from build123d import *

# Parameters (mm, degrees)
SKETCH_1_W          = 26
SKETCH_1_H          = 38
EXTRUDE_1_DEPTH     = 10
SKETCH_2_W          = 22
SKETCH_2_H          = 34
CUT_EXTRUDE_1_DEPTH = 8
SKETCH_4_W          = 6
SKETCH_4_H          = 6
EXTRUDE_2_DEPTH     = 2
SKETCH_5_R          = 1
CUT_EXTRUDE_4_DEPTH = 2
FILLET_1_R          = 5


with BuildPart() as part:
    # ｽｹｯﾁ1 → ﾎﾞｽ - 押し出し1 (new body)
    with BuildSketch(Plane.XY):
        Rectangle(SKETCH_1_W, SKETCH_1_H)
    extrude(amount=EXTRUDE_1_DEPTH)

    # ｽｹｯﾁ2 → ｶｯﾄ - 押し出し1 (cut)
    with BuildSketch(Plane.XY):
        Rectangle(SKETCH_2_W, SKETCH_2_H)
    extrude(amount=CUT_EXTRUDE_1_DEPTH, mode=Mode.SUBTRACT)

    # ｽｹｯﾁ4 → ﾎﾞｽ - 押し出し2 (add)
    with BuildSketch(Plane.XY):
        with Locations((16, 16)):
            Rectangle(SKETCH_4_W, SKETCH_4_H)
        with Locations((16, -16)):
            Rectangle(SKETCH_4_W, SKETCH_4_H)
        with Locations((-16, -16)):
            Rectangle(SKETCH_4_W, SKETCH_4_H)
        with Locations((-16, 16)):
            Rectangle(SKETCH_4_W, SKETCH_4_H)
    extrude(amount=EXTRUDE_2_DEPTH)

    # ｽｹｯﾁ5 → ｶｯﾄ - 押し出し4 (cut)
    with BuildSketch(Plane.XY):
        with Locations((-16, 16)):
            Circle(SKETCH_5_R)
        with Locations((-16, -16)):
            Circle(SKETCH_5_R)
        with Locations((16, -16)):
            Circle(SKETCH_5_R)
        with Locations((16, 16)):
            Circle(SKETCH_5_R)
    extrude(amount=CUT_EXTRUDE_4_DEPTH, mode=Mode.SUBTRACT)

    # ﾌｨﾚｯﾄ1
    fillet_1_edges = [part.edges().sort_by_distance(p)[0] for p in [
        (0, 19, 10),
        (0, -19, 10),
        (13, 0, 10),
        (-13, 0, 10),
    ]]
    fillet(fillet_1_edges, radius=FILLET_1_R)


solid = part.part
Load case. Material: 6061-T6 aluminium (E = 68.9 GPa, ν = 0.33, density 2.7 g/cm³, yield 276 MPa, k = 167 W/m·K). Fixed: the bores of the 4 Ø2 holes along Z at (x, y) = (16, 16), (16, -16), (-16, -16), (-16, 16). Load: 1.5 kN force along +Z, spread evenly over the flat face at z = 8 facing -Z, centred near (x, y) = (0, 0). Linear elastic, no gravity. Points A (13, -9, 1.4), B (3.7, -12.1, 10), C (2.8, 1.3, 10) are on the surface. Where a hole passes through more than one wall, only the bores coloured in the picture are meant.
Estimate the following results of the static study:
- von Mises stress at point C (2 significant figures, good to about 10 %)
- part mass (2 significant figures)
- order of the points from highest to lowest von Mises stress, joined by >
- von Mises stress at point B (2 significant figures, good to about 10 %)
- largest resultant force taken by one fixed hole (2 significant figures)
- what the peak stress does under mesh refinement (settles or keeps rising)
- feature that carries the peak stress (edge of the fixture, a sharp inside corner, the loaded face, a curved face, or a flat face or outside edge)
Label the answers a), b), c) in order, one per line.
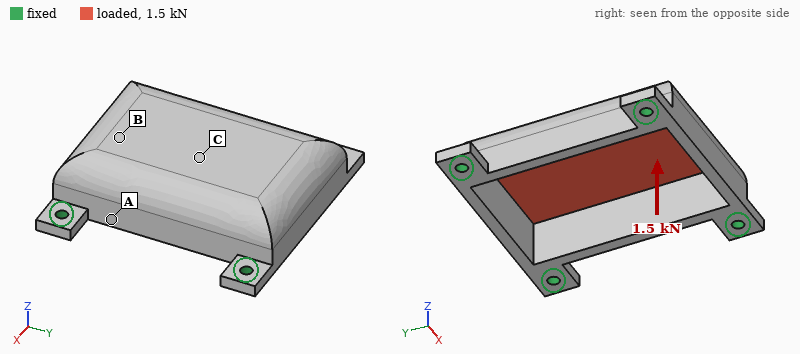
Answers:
a) 94 MPa
b) 9.5 g
c) C > B > A
d) 59 MPa
e) 450 N
f) keeps rising
g) edge of the fixture
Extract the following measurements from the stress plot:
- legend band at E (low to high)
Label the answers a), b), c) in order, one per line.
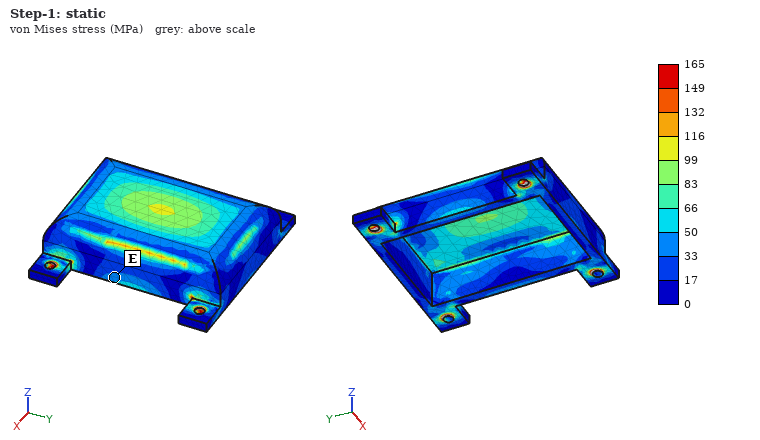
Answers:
a) 33 to 50 MPa
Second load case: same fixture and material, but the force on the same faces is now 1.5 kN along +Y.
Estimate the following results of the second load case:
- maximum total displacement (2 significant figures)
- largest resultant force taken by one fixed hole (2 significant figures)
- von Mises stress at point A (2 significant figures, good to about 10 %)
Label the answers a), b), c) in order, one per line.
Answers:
a) 22 µm
b) 410 N
c) 42 MPa
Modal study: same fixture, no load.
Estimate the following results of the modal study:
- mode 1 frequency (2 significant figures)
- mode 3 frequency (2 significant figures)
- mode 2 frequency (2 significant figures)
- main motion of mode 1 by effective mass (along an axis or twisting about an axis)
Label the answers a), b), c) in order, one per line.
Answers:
a) 12 kHz
b) 16 kHz
c) 15 kHz
d) along Z
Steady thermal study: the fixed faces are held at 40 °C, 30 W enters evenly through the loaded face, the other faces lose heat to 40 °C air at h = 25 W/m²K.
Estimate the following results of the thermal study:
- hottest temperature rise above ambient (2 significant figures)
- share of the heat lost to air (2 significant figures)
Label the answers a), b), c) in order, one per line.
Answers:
a) 33 K
b) 5.9 %
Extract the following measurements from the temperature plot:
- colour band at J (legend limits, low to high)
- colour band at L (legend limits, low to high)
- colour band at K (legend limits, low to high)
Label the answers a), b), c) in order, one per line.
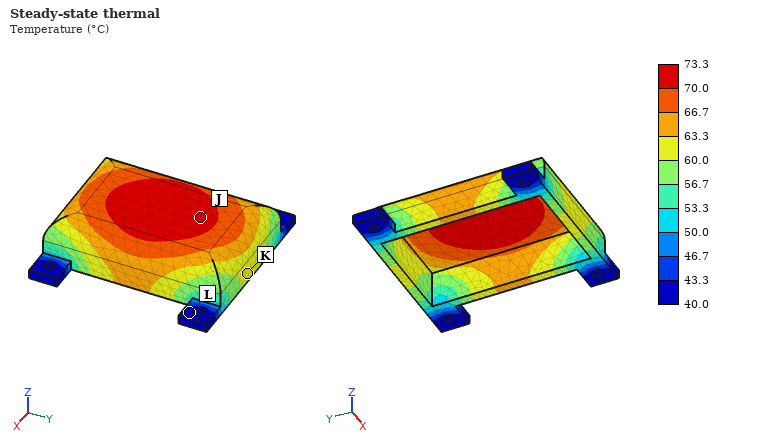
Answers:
a) 70.0 to 73.3 °C
b) 40.0 to 43.3 °C
c) 60.0 to 63.3 °C
